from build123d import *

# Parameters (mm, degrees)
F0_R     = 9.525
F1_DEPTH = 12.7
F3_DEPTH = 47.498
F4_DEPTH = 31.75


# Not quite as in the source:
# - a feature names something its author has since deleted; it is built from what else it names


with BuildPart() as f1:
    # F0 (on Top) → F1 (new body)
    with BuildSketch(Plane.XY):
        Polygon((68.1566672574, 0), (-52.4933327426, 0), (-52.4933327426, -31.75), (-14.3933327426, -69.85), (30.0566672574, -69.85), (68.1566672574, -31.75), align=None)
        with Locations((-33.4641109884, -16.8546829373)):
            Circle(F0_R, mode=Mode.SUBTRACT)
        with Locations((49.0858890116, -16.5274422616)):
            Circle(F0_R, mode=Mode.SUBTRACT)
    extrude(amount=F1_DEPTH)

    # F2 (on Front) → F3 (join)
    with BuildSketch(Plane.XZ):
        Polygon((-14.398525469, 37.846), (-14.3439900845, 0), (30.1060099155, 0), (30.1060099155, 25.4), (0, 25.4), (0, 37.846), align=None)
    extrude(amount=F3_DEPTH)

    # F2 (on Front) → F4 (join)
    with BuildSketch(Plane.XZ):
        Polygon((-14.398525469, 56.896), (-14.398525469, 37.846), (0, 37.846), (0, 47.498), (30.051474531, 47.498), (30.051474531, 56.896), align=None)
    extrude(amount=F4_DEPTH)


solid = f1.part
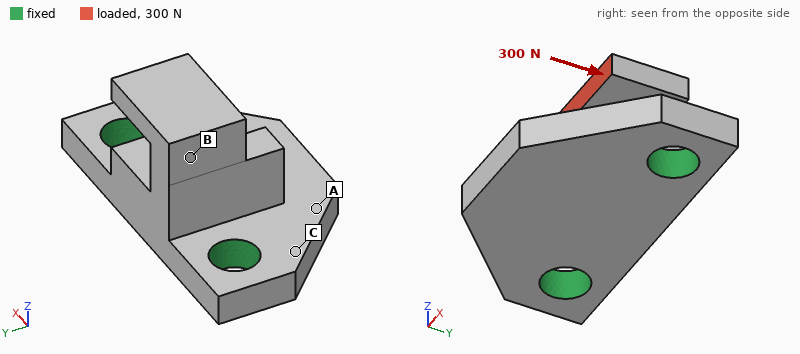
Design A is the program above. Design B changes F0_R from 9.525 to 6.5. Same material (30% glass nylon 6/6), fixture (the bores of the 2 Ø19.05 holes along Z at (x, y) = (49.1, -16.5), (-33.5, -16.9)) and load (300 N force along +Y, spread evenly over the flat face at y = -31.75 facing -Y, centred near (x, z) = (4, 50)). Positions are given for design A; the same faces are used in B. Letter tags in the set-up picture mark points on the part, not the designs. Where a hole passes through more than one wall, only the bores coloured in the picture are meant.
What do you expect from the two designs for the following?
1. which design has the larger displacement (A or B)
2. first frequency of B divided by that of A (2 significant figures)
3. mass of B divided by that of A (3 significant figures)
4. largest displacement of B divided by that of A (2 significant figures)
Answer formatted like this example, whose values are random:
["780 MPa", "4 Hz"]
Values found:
["B", "0.86", "1.03", "1.2"]
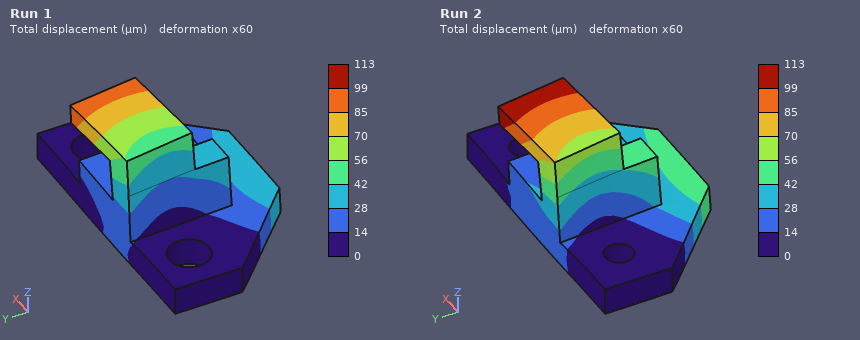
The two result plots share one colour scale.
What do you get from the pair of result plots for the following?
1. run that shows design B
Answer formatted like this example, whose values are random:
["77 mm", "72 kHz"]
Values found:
["Run 2"]
